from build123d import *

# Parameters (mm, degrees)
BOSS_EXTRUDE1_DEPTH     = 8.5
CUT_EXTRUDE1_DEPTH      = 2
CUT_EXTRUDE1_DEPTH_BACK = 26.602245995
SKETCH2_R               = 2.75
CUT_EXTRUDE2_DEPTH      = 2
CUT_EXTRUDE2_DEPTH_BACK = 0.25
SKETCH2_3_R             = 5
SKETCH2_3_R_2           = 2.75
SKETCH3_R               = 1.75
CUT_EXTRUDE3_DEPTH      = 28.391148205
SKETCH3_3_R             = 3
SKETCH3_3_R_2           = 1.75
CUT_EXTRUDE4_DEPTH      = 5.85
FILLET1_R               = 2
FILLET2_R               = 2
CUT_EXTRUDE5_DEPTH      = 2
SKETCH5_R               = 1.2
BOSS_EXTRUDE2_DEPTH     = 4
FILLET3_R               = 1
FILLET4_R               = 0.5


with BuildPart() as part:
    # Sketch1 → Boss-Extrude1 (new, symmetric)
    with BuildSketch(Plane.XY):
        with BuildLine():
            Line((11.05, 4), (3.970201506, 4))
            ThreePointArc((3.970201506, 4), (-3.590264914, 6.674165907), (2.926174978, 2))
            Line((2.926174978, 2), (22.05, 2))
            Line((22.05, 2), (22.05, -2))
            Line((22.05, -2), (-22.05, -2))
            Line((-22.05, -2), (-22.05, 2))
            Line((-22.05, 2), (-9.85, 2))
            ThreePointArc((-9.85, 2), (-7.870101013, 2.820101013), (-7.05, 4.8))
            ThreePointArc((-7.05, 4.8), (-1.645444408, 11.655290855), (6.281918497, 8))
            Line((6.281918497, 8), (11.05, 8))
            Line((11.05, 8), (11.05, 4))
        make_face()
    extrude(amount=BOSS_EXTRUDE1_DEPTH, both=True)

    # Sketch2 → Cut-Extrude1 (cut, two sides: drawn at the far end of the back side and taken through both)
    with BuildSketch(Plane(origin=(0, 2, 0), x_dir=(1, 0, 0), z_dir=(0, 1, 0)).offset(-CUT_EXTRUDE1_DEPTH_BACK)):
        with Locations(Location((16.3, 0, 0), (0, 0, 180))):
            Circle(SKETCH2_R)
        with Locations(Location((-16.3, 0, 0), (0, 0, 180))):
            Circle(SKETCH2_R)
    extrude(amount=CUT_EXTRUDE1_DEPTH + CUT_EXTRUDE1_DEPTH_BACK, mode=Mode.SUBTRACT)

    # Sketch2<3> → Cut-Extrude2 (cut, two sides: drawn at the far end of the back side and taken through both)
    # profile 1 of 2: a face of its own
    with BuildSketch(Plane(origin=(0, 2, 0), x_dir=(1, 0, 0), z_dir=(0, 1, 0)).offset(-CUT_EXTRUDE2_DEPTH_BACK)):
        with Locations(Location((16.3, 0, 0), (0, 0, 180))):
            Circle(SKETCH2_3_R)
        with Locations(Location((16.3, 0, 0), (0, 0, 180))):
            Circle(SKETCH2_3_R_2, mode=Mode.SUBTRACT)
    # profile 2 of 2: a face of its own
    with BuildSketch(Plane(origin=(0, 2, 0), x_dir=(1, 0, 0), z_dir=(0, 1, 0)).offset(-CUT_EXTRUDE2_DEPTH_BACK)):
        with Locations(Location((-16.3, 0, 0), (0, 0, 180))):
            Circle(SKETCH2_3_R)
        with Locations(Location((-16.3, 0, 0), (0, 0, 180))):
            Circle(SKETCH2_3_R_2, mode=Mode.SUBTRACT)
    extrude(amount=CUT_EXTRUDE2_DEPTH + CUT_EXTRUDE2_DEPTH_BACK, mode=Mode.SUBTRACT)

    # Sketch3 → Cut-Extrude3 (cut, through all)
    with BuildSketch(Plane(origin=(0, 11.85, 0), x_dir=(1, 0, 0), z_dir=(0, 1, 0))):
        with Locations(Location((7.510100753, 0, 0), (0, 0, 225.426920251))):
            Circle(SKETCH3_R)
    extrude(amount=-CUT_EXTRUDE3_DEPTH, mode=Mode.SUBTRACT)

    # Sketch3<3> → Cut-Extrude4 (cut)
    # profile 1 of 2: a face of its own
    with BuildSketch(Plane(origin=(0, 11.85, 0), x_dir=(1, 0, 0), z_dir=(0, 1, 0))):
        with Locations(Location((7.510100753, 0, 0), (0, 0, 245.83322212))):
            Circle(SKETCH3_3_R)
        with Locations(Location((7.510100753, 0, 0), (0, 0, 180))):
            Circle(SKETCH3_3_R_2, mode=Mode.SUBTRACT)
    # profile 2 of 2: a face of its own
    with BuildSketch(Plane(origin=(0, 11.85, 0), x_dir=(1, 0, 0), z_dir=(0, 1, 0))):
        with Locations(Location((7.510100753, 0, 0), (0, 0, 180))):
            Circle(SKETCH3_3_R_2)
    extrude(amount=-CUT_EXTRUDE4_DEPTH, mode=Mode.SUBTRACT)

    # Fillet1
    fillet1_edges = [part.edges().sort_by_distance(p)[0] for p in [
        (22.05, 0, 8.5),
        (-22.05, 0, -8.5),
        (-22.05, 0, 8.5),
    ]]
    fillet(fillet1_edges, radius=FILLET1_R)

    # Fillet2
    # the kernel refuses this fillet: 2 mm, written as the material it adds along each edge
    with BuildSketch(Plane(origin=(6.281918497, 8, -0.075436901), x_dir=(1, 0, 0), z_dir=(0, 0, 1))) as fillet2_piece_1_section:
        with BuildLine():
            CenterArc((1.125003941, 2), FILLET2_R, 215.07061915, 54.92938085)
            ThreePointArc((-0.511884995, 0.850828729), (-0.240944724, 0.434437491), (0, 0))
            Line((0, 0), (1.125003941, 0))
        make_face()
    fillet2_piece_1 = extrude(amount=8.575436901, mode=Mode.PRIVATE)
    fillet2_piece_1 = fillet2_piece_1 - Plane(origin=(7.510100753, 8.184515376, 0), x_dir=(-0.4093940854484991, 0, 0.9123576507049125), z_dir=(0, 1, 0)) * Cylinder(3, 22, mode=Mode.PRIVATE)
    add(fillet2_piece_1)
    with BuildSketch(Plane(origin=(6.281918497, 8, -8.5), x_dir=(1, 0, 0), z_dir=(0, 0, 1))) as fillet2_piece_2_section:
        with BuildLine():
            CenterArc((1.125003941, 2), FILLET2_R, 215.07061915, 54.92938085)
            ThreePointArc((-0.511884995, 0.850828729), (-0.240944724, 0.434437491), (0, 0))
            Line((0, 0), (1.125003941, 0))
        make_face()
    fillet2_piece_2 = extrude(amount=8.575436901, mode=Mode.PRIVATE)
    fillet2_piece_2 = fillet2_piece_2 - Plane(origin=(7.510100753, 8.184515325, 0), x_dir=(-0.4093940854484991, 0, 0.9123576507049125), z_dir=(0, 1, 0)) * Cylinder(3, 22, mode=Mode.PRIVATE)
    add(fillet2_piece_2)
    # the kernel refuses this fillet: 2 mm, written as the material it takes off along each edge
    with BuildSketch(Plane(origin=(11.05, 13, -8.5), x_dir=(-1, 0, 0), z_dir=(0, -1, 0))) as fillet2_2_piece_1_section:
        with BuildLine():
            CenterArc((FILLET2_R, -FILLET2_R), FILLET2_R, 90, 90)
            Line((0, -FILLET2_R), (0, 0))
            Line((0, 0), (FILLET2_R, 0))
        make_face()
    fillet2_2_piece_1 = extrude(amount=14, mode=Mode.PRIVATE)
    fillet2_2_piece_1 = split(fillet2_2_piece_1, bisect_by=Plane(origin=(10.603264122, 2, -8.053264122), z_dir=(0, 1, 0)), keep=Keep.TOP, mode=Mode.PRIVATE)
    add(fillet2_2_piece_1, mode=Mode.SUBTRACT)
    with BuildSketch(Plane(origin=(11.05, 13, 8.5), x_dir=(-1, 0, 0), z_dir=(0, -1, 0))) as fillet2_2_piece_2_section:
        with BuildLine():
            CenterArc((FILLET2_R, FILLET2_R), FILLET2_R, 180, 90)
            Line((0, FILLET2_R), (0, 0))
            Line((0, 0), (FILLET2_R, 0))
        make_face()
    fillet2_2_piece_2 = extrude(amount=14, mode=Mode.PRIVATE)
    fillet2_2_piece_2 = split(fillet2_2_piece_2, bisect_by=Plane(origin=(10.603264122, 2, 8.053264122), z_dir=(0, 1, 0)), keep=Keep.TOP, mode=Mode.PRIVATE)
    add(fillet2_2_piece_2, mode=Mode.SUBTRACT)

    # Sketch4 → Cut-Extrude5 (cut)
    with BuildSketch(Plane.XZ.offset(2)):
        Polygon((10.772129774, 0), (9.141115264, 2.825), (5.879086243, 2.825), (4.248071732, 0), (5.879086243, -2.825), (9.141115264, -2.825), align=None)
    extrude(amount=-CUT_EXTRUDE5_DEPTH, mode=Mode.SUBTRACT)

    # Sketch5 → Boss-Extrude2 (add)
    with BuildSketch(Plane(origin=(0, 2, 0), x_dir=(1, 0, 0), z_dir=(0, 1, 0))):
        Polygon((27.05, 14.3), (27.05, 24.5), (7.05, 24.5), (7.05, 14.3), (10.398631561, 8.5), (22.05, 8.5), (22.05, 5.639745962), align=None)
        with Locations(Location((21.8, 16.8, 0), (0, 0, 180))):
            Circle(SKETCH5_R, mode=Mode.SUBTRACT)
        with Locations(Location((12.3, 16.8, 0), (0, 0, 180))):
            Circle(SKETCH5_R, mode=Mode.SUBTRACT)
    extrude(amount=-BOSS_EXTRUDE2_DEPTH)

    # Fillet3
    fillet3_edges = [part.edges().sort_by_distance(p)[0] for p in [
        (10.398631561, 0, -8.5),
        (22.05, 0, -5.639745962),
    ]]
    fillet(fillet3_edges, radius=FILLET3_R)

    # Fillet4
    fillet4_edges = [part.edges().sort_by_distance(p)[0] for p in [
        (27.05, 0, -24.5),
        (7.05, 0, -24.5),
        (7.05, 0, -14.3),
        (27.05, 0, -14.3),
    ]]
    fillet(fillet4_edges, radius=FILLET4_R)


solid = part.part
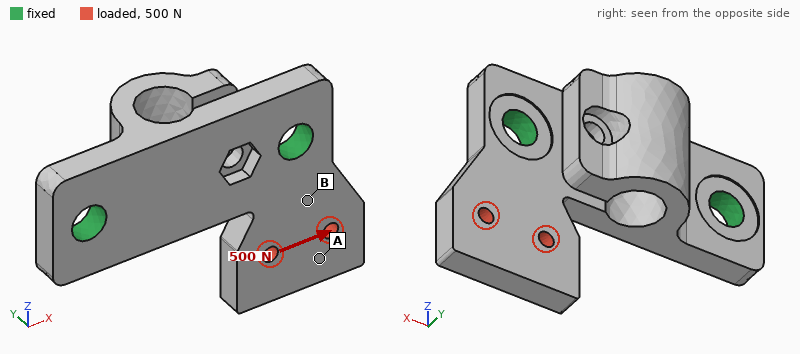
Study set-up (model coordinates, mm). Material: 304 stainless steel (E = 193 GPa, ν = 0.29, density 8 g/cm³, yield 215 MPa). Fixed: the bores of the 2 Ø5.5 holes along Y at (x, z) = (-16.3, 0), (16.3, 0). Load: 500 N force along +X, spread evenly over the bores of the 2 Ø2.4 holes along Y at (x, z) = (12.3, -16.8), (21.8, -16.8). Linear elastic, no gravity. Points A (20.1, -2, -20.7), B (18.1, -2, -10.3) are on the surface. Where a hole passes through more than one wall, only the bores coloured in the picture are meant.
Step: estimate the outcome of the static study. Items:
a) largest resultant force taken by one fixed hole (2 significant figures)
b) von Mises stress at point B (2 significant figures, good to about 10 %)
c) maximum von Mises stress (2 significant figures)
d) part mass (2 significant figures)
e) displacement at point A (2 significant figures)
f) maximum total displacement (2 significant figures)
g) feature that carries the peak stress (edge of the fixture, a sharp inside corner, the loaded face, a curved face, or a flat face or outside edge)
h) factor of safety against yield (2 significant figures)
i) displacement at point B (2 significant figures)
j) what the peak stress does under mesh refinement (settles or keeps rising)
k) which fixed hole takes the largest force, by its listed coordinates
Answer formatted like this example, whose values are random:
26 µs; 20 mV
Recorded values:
350 N; 22 MPa; 130 MPa; 41 g; 8.2 µm; 11 µm; a curved face; 1.7; 3.0 µm; settles; (16.3, 0)
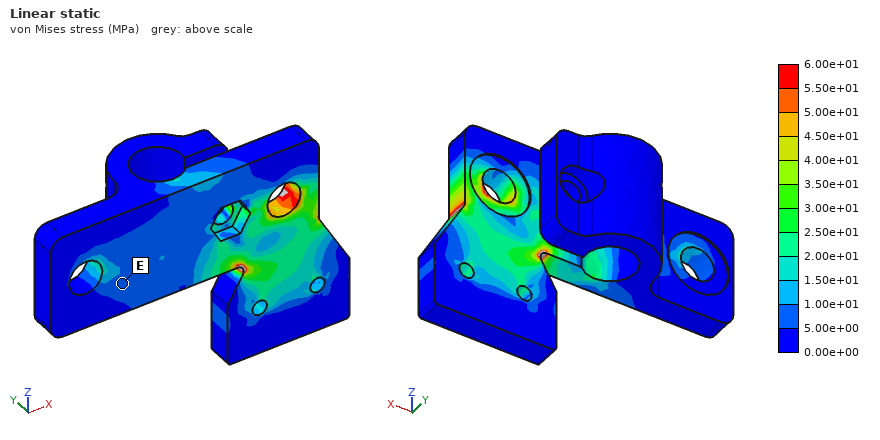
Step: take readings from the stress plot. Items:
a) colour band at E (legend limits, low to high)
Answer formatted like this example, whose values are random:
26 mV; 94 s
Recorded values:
5.00e+00 to 1.00e+01 MPa
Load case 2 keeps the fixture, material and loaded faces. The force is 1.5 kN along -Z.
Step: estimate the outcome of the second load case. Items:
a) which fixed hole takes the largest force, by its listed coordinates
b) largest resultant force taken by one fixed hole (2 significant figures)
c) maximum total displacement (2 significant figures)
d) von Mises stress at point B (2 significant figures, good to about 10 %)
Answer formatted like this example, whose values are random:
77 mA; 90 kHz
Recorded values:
(16.3, 0); 1.5 kN; 4.8 µm; 30 MPa
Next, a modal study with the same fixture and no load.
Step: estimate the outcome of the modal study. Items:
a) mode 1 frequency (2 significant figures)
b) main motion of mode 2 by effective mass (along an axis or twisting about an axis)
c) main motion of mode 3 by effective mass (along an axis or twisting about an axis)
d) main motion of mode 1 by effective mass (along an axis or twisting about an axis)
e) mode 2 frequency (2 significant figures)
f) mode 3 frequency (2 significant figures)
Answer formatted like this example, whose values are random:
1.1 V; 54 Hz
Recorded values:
4600 Hz; along Y; along Z; along Y; 5000 Hz; 7600 Hz
